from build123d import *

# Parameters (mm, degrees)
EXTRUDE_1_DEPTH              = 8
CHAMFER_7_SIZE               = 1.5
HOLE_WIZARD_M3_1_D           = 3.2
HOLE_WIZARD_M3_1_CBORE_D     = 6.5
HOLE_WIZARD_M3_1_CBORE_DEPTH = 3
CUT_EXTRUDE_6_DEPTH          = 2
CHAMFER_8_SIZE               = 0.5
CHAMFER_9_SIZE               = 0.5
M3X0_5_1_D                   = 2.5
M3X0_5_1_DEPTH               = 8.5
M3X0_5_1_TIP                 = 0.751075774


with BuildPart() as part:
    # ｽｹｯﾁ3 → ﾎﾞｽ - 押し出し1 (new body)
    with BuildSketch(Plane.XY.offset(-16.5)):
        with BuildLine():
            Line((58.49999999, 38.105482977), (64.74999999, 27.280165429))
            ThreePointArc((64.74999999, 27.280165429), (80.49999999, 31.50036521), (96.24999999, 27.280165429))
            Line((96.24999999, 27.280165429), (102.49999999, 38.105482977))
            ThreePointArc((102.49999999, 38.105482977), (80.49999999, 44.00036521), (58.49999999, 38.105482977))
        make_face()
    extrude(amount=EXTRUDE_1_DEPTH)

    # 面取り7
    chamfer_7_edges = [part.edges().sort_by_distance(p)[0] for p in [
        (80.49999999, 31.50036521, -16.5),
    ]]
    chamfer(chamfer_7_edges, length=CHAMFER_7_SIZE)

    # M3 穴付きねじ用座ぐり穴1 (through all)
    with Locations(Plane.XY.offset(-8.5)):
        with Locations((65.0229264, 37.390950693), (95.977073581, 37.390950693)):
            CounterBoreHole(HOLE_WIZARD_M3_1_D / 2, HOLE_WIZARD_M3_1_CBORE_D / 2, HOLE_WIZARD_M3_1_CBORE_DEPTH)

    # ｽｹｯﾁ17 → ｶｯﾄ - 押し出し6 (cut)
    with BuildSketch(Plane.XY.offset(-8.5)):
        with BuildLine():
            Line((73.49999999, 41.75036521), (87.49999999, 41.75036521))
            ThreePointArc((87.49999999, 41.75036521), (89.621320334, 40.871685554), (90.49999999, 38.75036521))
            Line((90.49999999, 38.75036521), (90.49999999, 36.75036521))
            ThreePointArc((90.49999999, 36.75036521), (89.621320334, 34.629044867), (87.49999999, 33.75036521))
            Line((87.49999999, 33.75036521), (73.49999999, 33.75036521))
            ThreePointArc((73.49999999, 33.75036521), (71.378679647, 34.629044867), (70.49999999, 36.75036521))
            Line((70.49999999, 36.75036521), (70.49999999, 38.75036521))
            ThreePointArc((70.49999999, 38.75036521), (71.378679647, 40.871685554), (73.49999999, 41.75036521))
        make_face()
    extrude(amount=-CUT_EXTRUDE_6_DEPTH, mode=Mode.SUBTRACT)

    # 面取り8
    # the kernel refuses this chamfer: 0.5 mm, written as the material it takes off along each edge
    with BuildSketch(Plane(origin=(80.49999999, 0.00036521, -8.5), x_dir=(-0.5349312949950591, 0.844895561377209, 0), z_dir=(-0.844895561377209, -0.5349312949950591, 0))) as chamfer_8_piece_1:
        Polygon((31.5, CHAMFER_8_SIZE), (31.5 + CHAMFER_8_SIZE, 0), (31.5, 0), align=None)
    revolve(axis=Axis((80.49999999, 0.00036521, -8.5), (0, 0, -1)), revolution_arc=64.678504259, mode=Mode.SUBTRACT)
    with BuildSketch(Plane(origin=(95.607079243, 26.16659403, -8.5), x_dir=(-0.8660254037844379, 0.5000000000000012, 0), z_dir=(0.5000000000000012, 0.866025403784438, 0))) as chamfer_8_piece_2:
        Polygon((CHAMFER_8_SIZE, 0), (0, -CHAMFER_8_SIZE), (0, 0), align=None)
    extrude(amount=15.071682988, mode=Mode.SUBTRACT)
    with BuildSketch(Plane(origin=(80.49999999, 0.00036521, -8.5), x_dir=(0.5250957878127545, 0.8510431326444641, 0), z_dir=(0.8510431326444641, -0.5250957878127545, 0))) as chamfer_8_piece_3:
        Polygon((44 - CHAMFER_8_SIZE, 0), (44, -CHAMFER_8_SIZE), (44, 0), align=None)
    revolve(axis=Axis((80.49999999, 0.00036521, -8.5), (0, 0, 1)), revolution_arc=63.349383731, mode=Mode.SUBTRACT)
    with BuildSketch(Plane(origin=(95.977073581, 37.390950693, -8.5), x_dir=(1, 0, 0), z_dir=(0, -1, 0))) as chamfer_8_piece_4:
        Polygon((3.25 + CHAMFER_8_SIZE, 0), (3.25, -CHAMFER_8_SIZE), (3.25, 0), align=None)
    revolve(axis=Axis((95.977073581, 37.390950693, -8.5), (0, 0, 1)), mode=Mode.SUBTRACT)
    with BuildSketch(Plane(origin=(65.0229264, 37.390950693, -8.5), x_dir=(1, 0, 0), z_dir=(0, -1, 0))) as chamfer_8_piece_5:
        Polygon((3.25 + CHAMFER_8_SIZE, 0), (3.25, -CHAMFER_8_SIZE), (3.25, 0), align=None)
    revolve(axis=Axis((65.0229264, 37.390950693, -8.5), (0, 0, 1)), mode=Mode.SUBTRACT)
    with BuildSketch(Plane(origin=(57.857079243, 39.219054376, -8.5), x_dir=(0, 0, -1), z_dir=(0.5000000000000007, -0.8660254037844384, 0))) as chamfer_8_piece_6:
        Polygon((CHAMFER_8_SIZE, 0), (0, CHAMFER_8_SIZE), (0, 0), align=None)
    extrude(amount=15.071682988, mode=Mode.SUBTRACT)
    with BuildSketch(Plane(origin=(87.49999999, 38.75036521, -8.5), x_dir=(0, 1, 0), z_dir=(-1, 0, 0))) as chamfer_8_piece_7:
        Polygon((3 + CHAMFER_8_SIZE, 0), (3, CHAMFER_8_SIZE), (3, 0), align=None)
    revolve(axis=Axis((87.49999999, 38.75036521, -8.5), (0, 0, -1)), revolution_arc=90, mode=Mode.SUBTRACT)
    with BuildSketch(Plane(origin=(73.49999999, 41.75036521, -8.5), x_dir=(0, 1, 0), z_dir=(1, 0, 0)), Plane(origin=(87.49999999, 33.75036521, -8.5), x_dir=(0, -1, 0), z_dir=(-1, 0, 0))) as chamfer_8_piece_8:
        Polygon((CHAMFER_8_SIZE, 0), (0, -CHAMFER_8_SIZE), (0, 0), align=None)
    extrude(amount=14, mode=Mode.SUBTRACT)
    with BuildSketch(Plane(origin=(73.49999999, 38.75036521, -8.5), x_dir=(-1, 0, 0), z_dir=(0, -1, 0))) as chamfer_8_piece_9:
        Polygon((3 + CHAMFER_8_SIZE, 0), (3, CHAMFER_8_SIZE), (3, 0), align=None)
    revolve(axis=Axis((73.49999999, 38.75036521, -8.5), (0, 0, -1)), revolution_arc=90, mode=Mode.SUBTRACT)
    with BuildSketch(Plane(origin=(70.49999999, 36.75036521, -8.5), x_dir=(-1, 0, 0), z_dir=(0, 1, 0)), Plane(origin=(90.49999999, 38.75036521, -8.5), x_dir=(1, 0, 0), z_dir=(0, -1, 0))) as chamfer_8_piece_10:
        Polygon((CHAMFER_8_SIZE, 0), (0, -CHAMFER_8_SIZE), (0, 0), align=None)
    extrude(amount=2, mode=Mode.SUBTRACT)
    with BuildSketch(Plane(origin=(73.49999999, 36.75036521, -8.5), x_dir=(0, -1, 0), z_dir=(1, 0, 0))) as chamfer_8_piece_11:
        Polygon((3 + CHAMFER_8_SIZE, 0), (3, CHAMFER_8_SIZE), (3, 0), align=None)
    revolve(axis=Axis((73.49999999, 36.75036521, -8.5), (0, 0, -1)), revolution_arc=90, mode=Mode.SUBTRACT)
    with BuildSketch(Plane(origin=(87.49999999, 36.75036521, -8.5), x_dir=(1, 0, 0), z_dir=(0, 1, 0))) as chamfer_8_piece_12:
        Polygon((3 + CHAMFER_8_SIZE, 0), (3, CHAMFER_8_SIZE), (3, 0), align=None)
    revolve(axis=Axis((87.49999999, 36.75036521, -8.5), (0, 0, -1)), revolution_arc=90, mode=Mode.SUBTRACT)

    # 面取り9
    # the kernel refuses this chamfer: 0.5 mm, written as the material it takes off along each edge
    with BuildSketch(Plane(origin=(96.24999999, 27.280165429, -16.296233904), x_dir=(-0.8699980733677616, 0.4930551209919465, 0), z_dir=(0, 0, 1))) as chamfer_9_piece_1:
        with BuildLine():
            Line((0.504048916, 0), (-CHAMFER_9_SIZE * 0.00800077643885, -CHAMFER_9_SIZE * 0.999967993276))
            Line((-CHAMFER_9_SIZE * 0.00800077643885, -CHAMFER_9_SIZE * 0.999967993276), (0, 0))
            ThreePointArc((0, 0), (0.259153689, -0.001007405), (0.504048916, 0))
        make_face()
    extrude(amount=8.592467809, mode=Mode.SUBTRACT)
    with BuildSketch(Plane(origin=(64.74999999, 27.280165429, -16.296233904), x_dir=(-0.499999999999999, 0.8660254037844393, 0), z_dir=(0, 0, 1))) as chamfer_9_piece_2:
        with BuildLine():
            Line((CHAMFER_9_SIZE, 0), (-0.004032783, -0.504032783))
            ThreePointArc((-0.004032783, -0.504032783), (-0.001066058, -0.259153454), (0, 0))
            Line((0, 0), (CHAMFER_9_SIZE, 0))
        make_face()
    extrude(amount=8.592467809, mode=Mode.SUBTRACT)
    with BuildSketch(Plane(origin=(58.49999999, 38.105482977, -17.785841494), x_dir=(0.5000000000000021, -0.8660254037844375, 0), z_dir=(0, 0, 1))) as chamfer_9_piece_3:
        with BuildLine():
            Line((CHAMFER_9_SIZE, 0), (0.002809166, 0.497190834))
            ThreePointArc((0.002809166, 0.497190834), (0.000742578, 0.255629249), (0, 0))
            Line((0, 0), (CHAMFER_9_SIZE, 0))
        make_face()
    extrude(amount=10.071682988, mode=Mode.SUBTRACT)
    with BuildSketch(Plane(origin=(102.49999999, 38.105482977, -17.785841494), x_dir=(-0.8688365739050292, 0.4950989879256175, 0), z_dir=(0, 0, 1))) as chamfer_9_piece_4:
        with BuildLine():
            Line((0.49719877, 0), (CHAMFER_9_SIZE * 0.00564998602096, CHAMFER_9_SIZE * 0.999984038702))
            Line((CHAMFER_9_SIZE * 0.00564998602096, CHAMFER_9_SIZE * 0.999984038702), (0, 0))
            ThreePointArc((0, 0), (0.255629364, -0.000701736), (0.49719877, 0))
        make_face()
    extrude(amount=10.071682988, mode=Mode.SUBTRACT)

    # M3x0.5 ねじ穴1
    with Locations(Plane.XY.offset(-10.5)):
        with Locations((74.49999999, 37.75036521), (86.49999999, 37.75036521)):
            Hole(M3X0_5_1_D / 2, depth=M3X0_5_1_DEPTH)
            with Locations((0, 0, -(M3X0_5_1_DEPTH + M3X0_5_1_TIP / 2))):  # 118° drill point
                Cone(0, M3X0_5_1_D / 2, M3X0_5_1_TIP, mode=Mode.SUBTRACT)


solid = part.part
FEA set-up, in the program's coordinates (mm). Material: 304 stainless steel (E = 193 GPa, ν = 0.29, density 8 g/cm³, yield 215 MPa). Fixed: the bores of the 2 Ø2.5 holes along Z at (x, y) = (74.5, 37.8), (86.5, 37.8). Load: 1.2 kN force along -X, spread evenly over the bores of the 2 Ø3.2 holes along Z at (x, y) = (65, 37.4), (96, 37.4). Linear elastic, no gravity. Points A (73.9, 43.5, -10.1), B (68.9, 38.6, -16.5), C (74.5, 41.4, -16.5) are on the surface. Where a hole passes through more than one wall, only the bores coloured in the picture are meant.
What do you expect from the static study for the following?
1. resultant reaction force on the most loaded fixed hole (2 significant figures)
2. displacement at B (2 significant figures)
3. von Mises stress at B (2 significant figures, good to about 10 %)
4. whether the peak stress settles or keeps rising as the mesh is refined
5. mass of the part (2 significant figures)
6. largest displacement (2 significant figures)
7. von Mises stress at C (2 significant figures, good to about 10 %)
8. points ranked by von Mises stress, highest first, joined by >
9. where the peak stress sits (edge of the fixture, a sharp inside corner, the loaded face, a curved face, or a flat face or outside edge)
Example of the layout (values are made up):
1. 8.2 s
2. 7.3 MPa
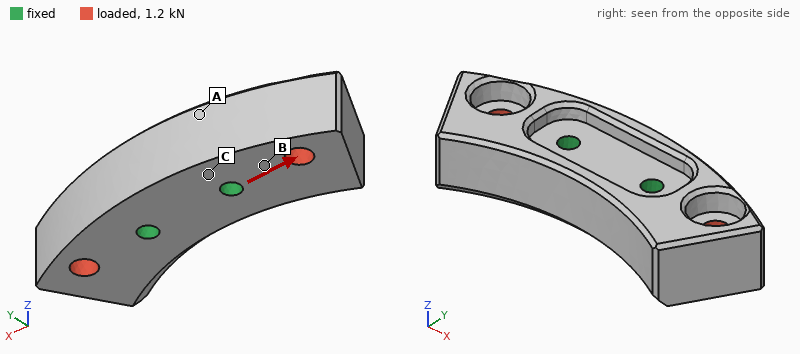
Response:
1. 600 N
2. 0.51 µm
3. 18 MPa
4. keeps rising
5. 26 g
6. 1.3 µm
7. 6.0 MPa
8. B > C > A
9. edge of the fixture
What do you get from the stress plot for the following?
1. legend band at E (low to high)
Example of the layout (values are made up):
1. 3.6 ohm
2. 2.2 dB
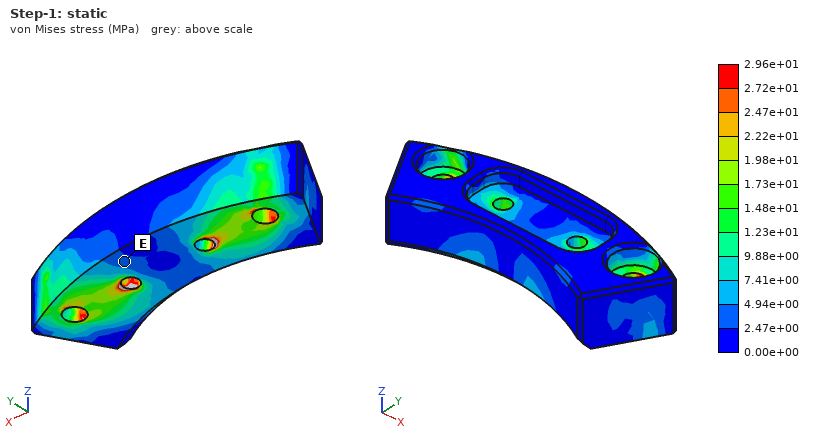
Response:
1. 2.47e+00 to 4.94e+00 MPa
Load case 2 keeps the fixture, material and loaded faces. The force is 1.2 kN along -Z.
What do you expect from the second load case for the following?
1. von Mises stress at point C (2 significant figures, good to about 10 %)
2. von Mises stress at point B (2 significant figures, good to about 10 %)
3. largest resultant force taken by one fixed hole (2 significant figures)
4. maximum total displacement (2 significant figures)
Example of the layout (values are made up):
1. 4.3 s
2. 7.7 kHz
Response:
1. 30 MPa
2. 32 MPa
3. 620 N
4. 9.2 µm
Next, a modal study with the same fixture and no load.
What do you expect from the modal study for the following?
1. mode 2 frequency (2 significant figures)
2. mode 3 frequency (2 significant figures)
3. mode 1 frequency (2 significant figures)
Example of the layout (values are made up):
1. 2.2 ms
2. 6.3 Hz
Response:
1. 21 kHz
2. 24 kHz
3. 20 kHz
